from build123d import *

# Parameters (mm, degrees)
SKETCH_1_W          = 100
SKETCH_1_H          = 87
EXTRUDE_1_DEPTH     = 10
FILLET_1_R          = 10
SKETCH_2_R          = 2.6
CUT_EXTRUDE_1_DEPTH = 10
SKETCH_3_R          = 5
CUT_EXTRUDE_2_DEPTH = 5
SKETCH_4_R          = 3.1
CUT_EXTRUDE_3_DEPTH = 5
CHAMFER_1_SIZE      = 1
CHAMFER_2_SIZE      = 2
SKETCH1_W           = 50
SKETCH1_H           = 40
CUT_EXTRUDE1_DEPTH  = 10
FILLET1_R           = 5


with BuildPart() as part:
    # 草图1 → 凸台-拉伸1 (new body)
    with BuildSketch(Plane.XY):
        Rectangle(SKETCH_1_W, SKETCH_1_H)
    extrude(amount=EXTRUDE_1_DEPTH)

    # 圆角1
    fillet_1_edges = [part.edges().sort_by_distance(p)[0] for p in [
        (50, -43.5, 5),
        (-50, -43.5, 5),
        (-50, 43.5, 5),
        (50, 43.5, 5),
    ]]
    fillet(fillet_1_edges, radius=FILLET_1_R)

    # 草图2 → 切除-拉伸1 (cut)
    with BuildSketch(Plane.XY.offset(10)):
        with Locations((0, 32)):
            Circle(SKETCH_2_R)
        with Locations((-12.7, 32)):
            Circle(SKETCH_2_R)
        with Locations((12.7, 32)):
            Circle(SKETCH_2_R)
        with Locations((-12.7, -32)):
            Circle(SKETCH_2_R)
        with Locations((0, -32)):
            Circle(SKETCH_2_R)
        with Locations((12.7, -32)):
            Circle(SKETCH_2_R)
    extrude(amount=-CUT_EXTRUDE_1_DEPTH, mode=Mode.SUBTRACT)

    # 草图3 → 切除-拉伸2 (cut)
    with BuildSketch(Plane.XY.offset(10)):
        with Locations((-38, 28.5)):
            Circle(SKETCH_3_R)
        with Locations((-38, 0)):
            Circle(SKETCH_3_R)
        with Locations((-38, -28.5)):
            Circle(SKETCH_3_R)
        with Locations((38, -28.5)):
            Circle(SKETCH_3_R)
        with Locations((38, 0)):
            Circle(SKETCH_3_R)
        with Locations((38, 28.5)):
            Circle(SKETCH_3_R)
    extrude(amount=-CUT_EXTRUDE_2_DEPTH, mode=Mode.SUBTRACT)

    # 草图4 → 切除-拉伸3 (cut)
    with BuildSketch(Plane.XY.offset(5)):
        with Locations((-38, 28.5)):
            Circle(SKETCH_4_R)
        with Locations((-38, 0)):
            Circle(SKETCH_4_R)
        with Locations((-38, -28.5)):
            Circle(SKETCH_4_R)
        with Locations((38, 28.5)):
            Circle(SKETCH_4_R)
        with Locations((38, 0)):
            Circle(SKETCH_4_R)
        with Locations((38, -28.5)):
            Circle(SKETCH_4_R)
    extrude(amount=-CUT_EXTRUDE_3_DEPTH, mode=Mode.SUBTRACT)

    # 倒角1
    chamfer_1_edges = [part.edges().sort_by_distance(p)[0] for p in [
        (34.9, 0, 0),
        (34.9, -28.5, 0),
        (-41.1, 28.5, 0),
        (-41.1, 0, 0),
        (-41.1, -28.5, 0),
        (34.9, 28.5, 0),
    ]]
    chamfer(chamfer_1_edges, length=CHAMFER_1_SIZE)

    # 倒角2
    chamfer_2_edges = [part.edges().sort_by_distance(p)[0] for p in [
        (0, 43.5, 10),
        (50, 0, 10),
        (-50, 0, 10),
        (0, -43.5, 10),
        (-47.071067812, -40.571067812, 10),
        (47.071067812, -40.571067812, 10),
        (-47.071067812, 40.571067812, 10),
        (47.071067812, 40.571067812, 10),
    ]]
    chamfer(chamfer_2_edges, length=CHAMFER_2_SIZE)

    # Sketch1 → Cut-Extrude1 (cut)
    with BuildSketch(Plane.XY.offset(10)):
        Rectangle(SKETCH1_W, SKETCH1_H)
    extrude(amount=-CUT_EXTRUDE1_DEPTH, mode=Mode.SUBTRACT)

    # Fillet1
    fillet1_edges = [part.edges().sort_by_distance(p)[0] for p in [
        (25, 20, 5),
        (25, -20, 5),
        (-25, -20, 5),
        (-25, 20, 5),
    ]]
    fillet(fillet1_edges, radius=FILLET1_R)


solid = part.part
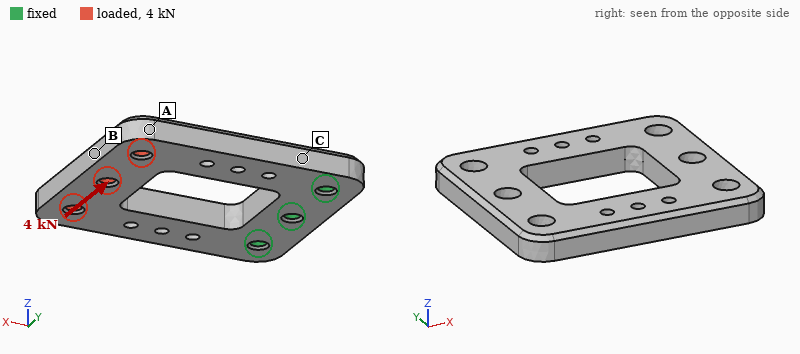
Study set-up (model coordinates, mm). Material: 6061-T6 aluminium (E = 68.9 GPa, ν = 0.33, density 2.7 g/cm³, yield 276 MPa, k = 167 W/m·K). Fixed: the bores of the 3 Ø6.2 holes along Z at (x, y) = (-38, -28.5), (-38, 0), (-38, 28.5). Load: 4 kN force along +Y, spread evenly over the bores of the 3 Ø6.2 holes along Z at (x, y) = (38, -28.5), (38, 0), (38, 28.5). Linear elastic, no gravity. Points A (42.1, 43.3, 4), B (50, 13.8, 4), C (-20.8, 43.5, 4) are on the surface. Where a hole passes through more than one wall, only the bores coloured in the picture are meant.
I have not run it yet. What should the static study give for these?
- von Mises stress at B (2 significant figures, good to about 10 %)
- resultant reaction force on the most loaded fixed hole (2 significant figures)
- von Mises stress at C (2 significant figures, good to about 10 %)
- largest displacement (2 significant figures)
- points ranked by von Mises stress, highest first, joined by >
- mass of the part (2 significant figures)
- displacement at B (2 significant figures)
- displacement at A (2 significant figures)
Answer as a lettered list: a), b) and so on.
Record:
a) 32 MPa
b) 4.9 kN
c) 62 MPa
d) 0.22 mm
e) C > B > A
f) 160 g
g) 0.19 mm
h) 0.21 mm
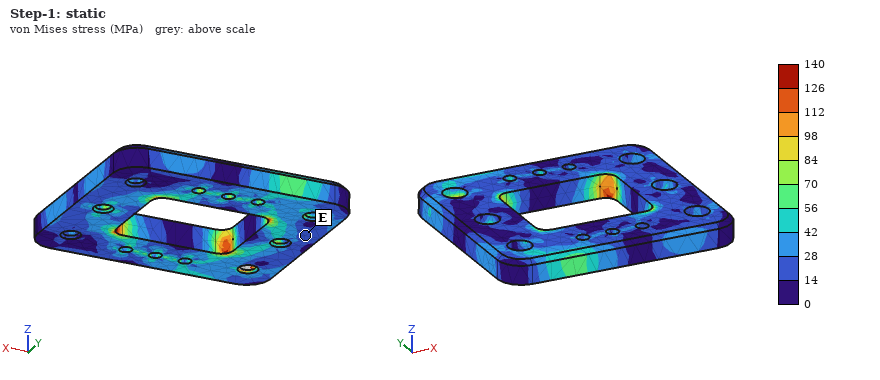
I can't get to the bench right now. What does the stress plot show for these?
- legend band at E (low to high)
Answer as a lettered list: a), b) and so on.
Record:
a) 14 to 28 MPa
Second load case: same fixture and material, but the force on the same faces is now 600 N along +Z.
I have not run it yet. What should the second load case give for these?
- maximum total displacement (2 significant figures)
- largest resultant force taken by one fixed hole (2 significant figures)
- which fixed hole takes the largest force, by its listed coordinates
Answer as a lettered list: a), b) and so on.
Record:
a) 0.58 mm
b) 380 N
c) (-38, 0)
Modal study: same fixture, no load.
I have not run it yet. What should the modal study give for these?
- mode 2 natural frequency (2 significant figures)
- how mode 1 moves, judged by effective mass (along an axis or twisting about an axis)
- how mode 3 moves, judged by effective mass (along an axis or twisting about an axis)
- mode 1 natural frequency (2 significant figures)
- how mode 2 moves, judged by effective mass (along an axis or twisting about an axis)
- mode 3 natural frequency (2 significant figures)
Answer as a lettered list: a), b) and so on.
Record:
a) 1800 Hz
b) along Z
c) along Y
d) 710 Hz
e) twisting about X
f) 2900 Hz
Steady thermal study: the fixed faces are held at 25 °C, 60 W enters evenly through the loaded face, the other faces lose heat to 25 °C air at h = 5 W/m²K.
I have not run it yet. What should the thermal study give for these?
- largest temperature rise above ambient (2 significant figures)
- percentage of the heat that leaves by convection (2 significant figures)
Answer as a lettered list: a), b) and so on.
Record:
a) 67 K
b) 5.1 %
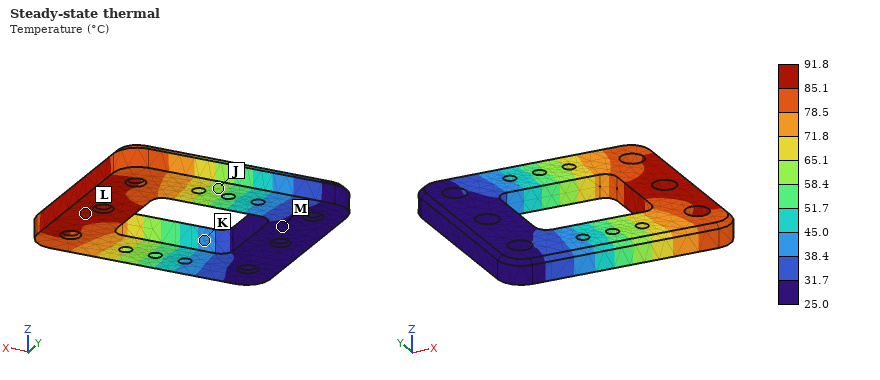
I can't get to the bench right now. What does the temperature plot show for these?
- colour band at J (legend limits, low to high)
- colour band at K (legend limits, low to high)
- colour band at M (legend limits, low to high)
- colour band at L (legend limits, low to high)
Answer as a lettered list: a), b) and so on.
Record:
a) 58.4 to 65.1 °C
b) 38.4 to 45.0 °C
c) 25.0 to 31.7 °C
d) 85.1 to 91.8 °C
